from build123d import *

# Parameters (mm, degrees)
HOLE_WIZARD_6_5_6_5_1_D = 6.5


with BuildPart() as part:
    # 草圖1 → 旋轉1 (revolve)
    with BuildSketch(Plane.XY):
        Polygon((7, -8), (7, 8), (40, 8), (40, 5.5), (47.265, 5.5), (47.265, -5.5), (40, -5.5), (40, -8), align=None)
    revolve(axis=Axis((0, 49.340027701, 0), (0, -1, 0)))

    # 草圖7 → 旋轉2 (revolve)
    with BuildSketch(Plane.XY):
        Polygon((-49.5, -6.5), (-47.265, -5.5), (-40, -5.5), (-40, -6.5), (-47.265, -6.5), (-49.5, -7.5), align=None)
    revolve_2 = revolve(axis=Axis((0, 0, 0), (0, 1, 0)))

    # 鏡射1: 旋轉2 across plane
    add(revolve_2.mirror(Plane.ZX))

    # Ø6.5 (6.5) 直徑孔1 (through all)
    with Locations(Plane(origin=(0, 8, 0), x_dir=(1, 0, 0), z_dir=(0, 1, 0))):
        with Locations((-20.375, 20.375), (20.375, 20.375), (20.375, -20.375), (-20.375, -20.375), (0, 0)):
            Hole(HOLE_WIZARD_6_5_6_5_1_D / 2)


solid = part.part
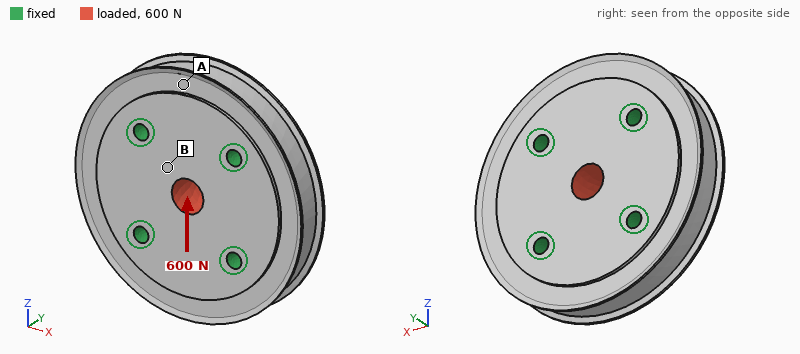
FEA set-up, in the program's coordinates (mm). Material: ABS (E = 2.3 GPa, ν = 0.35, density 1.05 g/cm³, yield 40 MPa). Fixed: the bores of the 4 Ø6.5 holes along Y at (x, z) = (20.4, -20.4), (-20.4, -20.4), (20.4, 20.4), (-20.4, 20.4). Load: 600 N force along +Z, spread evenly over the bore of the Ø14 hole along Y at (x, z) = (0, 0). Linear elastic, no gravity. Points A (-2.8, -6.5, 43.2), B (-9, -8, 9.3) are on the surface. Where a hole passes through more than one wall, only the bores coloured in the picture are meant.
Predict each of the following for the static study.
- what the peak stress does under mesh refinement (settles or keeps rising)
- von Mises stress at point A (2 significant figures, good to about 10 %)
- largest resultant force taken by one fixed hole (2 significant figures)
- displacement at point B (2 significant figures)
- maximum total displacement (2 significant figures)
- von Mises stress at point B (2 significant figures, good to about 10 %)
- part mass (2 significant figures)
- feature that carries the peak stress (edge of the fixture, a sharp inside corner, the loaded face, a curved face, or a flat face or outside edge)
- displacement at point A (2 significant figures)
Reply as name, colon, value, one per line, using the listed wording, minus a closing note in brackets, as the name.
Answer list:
what the peak stress does under mesh refinement: keeps rising
von Mises stress at point A: 0.16 MPa
largest resultant force taken by one fixed hole: 160 N
displacement at point B: 4.5 µm
maximum total displacement: 8.0 µm
von Mises stress at point B: 0.65 MPa
part mass: 110 g
feature that carries the peak stress: edge of the fixture
displacement at point A: 2.6 µm
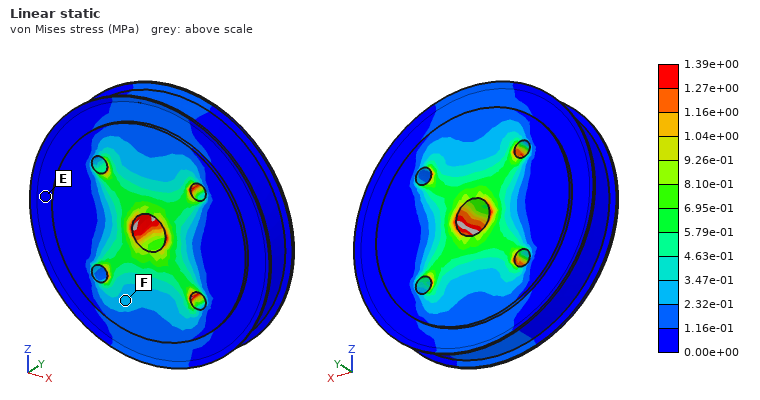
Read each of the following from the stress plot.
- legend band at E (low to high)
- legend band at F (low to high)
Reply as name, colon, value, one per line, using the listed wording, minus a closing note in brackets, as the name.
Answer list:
legend band at E: 0.00e+00 to 1.16e-01 MPa
legend band at F: 2.32e-01 to 3.47e-01 MPa
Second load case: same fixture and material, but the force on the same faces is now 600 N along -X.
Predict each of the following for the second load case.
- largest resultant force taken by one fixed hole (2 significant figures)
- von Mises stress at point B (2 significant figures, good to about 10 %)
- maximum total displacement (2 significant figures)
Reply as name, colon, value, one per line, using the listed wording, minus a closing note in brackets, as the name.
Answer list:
largest resultant force taken by one fixed hole: 160 N
von Mises stress at point B: 0.64 MPa
maximum total displacement: 8.0 µm
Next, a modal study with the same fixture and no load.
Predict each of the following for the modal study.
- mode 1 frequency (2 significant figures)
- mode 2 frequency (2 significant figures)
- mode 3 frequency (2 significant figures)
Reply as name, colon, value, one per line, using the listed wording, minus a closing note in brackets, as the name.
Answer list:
mode 1 frequency: 4200 Hz
mode 2 frequency: 4600 Hz
mode 3 frequency: 4600 Hz
